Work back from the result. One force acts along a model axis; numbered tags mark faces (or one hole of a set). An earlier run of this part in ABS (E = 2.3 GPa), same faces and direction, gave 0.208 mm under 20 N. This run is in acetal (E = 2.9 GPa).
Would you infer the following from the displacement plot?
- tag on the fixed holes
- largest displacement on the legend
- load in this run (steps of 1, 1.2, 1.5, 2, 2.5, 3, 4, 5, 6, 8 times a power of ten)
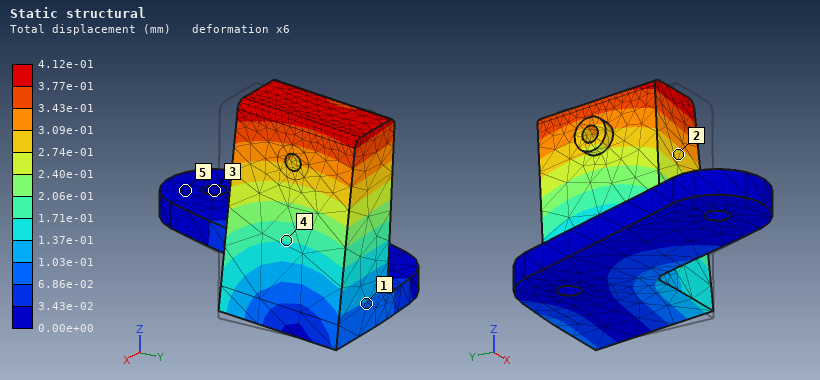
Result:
3
4.12e-01 mm
50 N
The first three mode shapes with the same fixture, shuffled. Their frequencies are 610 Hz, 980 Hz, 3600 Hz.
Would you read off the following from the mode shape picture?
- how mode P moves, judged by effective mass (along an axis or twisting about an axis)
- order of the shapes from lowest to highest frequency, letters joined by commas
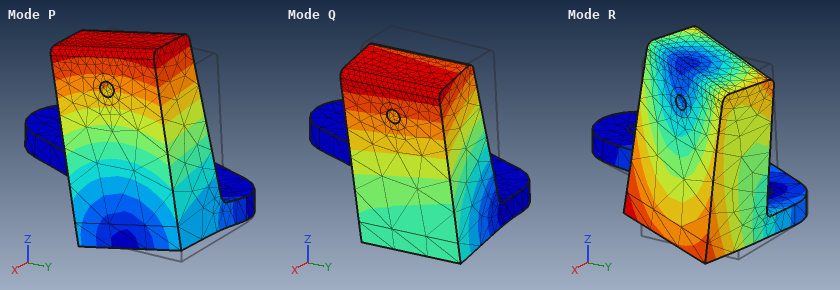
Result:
along Y
Q, P, R
